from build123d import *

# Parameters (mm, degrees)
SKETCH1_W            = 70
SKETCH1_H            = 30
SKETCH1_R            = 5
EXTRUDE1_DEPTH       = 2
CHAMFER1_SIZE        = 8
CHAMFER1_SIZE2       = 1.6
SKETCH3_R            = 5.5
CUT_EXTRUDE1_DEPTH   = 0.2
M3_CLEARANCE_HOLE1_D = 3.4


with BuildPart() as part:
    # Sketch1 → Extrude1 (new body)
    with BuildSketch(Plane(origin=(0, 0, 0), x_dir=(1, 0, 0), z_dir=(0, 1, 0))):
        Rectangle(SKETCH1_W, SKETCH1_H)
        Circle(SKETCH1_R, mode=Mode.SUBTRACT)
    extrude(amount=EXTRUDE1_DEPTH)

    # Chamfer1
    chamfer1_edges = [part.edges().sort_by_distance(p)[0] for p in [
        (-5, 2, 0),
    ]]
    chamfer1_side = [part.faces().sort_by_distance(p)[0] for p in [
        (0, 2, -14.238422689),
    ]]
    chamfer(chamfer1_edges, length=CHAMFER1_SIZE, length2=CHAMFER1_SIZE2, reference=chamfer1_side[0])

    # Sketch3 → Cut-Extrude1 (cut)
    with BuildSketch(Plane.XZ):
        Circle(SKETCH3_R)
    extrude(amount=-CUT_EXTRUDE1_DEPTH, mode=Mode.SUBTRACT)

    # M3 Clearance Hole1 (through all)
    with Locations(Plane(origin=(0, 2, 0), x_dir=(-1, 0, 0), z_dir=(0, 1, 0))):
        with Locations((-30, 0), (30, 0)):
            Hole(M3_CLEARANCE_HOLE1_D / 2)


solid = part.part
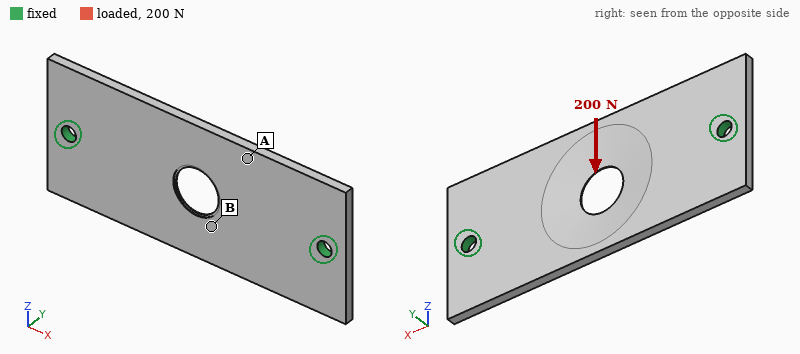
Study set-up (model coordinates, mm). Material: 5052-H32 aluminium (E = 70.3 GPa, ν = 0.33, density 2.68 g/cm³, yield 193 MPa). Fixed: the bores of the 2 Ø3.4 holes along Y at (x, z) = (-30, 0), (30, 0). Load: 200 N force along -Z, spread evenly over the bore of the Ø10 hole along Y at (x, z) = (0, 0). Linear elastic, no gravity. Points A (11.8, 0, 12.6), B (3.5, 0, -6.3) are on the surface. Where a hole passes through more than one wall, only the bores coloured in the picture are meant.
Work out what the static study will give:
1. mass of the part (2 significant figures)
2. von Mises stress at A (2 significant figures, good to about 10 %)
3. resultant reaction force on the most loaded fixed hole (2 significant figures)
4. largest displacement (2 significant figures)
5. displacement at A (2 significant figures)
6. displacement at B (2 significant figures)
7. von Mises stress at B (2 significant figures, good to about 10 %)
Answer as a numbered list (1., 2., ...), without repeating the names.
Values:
1. 9.9 g
2. 5.7 MPa
3. 100 N
4. 14 µm
5. 9.6 µm
6. 7.7 µm
7. 11 MPa
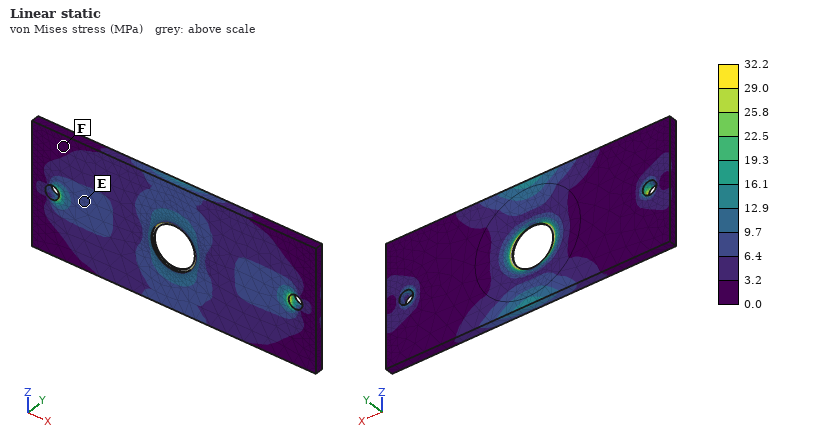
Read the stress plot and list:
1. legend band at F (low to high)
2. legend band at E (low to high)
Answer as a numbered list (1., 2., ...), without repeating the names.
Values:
1. 0.0 to 3.2 MPa
2. 6.4 to 9.7 MPa
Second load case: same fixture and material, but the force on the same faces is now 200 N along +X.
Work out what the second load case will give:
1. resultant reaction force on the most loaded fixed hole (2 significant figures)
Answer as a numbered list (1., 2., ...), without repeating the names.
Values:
1. 100 N
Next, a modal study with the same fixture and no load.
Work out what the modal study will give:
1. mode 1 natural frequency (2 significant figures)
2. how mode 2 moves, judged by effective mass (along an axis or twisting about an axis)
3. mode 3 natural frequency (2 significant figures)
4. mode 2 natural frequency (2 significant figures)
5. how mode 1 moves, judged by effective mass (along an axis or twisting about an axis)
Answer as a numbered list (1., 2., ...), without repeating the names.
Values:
1. 2700 Hz
2. twisting about X
3. 6000 Hz
4. 3200 Hz
5. along Y
